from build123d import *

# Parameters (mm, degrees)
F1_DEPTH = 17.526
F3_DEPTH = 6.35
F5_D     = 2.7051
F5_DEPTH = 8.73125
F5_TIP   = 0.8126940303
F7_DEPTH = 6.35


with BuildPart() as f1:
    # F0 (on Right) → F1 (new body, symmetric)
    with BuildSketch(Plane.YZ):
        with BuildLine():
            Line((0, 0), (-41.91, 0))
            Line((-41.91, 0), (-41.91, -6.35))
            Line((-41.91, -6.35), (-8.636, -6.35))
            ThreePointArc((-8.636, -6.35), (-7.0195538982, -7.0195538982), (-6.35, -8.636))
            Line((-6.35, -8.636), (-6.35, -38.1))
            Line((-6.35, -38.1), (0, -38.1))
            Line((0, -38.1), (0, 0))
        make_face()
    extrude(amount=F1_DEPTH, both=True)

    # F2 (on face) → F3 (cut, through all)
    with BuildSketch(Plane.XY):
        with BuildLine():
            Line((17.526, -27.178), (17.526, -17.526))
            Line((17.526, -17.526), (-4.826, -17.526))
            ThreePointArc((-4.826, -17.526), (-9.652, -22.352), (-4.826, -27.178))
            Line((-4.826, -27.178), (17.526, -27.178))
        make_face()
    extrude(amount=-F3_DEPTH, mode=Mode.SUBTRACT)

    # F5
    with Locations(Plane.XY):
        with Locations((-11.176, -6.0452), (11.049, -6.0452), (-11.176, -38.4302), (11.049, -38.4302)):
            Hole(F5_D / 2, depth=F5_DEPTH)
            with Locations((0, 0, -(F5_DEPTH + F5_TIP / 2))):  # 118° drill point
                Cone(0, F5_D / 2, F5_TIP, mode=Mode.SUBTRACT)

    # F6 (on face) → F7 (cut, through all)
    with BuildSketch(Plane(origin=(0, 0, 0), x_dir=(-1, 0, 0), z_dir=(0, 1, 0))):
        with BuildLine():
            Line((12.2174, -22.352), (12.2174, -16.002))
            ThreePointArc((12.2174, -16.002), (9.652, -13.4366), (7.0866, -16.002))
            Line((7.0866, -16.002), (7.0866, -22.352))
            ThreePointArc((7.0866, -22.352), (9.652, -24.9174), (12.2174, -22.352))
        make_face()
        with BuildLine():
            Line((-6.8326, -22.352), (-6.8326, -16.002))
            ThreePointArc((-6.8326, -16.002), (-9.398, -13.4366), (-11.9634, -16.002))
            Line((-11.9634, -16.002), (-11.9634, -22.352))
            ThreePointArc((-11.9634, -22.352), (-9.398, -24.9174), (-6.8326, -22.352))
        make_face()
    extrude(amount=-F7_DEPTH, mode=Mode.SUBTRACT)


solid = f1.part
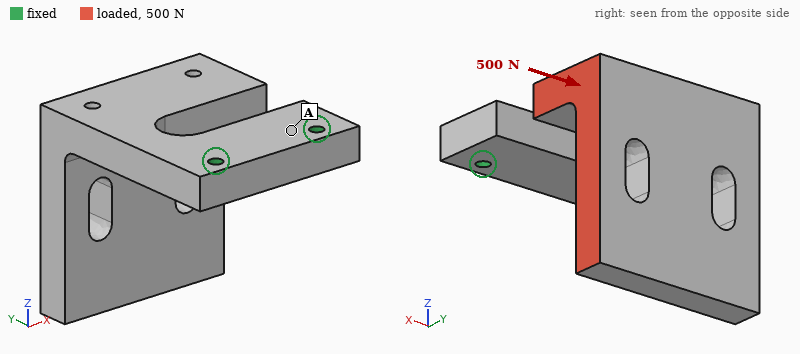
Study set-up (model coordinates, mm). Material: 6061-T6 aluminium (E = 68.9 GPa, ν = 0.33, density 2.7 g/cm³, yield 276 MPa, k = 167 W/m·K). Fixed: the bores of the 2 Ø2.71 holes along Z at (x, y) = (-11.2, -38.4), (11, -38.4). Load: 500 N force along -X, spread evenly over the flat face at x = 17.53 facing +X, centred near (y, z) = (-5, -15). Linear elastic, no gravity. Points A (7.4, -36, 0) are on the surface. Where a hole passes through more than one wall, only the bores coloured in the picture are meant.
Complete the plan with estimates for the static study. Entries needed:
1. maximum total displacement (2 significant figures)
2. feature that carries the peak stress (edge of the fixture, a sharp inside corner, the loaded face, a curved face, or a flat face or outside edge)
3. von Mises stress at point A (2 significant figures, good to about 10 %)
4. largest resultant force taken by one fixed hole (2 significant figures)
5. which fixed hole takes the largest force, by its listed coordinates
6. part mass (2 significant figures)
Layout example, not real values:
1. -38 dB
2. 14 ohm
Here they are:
1. 0.71 mm
2. a curved face
3. 32 MPa
4. 1.0 kN
5. (11, -38.4)
6. 38 g
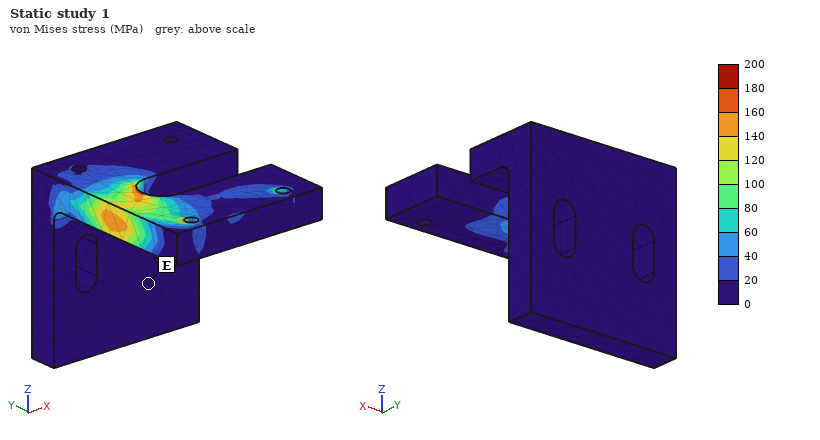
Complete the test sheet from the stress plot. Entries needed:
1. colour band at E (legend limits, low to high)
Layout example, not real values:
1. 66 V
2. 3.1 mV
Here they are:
1. 0 to 20 MPa
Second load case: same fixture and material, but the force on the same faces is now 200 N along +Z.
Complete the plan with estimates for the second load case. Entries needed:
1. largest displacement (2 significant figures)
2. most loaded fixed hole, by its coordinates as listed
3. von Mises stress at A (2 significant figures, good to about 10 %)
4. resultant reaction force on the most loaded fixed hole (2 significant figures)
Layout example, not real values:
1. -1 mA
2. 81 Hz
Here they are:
1. 0.71 mm
2. (11, -38.4)
3. 27 MPa
4. 160 N
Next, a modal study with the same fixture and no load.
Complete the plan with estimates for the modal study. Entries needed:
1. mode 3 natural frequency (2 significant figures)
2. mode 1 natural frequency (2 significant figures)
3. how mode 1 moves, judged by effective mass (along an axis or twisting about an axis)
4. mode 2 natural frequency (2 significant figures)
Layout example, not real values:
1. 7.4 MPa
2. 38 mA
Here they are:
1. 2000 Hz
2. 740 Hz
3. along Z
4. 970 Hz
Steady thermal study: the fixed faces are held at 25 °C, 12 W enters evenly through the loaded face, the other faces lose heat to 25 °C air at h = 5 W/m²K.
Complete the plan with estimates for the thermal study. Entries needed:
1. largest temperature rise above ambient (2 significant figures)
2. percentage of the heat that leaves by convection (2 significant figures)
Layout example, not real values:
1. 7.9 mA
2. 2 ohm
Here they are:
1. 40 K
2. 6.4 %
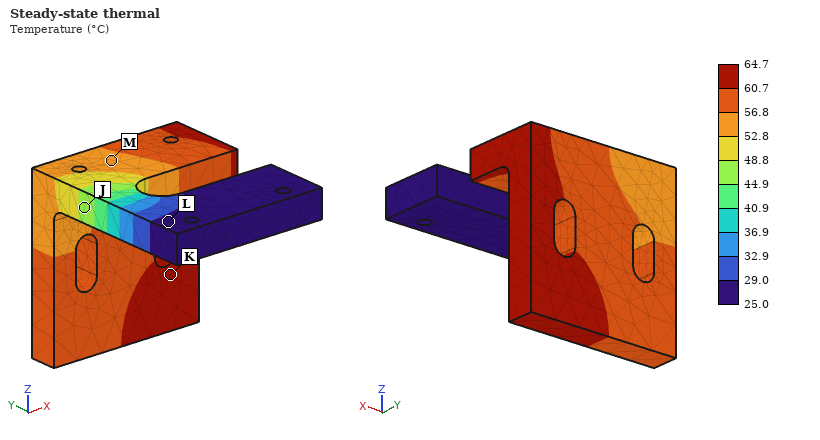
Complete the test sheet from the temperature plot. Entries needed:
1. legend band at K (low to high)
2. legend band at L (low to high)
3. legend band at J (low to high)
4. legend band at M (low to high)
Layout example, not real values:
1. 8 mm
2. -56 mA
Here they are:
1. 60.7 to 64.7 °C
2. 25.0 to 29.0 °C
3. 44.9 to 48.8 °C
4. 52.8 to 56.8 °C
